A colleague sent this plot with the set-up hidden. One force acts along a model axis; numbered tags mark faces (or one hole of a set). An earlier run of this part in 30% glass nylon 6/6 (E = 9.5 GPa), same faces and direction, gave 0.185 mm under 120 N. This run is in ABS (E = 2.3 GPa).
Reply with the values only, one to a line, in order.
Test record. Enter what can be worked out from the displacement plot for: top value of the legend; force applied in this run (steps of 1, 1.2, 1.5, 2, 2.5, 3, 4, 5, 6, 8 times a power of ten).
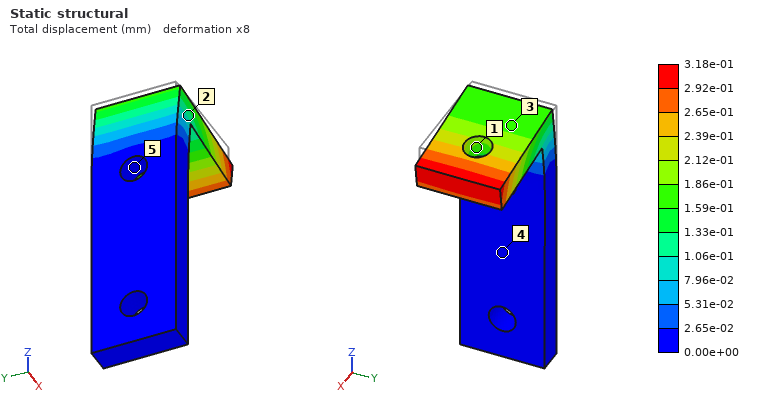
3.18e-01 mm
50 N
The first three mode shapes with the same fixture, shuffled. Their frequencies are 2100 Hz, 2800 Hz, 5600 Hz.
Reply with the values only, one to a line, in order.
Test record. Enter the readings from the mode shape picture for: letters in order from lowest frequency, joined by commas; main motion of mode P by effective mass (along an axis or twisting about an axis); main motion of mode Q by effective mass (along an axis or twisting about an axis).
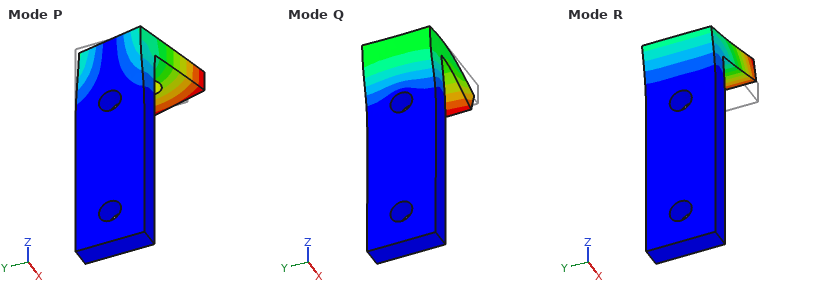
R, P, Q
along Y
along X
